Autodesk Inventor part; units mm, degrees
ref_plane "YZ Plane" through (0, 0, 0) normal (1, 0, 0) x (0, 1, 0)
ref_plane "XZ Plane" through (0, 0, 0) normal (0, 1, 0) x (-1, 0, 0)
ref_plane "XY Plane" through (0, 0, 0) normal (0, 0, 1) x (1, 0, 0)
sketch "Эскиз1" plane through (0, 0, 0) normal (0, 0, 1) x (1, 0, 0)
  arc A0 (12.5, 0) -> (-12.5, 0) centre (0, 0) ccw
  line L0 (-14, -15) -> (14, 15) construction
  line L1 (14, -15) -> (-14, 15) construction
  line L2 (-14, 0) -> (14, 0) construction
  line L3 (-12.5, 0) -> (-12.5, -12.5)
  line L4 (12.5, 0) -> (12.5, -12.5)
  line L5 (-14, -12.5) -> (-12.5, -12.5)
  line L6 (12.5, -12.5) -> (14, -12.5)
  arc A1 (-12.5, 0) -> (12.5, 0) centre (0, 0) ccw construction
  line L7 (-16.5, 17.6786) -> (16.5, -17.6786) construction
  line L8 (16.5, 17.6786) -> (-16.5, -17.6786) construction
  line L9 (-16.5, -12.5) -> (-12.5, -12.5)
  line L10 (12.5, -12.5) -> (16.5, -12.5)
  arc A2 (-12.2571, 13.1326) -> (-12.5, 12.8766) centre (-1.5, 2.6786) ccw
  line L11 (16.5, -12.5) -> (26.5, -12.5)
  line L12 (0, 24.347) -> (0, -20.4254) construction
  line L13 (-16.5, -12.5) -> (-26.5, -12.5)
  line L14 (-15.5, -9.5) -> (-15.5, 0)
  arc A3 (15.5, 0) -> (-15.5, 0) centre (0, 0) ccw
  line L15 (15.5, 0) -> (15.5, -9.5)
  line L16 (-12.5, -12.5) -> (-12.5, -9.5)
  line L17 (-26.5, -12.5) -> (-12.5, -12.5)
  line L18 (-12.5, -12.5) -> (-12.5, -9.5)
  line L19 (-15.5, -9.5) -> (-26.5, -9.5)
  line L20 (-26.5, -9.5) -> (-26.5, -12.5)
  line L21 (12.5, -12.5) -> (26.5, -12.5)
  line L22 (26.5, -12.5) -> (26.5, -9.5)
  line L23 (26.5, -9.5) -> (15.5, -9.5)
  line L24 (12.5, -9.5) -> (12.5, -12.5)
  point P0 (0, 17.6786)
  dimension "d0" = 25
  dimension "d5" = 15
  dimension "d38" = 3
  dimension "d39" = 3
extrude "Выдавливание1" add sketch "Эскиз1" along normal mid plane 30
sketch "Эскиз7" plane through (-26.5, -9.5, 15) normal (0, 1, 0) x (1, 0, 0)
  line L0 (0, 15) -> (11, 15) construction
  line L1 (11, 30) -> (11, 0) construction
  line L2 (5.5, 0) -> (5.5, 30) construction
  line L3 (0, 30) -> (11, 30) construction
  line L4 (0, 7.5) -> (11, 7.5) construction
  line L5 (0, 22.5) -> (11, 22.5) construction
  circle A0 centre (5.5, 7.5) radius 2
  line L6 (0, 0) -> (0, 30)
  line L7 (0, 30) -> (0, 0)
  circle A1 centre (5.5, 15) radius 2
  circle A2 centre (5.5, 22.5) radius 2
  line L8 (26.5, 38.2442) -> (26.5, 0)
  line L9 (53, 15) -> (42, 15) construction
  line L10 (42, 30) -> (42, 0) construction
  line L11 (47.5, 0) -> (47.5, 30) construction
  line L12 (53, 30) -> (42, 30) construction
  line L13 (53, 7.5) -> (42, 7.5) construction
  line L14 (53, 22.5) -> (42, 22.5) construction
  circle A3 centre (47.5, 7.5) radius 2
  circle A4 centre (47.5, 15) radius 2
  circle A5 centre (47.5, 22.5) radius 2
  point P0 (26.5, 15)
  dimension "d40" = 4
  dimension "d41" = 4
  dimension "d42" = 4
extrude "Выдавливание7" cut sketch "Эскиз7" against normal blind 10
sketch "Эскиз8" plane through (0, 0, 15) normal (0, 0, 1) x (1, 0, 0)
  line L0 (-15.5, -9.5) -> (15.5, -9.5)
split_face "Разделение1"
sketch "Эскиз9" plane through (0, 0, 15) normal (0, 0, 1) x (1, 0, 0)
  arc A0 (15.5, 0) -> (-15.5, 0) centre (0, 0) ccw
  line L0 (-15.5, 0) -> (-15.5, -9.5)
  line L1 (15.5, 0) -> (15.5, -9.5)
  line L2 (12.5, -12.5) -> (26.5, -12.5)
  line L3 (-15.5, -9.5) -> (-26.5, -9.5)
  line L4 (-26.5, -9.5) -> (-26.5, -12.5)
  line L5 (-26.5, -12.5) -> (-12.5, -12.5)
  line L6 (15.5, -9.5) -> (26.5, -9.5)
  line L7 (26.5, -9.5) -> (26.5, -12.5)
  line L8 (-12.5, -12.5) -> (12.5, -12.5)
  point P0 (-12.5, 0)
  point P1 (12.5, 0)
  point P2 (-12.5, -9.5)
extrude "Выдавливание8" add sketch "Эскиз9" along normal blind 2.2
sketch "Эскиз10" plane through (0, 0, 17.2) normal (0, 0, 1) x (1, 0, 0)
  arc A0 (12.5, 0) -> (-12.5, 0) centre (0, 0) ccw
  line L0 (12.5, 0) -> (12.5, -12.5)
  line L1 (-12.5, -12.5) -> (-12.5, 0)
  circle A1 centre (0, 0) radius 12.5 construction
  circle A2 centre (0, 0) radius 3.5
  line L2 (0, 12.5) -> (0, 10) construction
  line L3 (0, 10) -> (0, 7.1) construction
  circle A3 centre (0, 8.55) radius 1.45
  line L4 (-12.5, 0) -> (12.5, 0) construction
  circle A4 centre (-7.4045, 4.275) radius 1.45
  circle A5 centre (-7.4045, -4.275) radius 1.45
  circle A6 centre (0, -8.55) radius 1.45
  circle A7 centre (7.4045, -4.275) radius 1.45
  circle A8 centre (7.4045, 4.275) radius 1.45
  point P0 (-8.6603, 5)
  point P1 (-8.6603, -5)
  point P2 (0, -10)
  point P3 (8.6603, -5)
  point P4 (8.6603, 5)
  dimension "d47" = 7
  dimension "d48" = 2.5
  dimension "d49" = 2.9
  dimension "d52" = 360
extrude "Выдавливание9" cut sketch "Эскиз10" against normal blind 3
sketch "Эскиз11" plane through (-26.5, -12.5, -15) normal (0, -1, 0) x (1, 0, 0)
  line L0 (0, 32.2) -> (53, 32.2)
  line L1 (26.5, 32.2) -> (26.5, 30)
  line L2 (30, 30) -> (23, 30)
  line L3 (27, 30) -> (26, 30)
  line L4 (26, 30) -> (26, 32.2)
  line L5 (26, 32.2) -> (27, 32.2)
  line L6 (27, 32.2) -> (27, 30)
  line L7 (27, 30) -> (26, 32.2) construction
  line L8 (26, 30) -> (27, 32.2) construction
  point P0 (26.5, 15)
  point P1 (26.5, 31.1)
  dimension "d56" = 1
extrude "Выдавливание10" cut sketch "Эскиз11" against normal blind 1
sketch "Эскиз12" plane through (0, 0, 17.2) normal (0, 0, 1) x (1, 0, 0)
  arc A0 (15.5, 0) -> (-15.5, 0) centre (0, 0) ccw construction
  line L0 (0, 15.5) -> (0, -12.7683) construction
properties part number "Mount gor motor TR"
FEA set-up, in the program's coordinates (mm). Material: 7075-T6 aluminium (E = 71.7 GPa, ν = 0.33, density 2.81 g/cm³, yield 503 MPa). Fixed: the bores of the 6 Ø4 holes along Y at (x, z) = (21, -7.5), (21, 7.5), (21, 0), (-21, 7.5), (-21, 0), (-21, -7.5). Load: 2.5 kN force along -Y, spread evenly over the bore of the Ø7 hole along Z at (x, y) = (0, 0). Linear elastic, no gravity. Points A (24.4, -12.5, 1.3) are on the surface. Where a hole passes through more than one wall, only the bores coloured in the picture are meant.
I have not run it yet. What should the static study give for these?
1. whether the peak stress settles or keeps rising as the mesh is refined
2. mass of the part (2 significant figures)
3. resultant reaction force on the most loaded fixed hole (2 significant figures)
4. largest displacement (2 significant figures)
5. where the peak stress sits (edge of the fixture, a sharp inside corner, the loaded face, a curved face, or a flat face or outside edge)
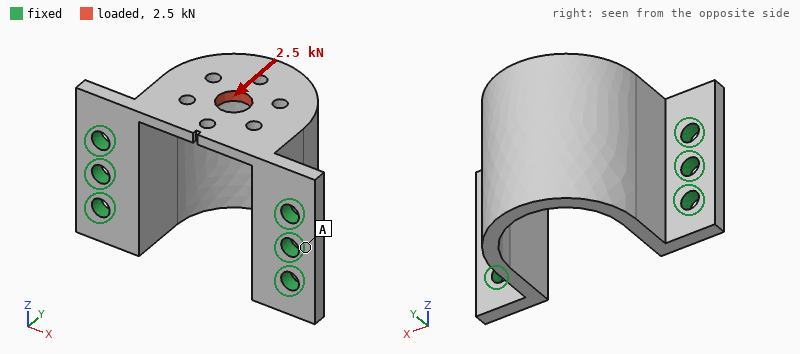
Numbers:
keeps rising
27 g
1.7 kN
0.11 mm
edge of the fixture
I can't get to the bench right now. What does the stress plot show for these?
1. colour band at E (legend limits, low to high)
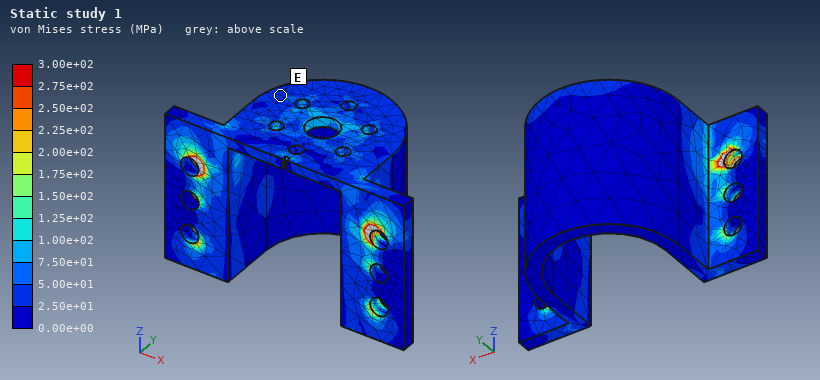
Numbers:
2.50e+01 to 5.00e+01 MPa
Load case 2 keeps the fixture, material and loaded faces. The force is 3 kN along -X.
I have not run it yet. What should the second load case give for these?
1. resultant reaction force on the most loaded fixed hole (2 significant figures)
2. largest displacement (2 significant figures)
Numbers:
1.7 kN
56 µm
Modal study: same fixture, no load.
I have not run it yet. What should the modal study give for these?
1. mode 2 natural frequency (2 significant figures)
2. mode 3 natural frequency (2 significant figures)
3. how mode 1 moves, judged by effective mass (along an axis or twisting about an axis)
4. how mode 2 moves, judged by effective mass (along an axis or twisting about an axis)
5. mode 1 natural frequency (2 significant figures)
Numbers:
6200 Hz
14 kHz
along X
along Z
5500 Hz
